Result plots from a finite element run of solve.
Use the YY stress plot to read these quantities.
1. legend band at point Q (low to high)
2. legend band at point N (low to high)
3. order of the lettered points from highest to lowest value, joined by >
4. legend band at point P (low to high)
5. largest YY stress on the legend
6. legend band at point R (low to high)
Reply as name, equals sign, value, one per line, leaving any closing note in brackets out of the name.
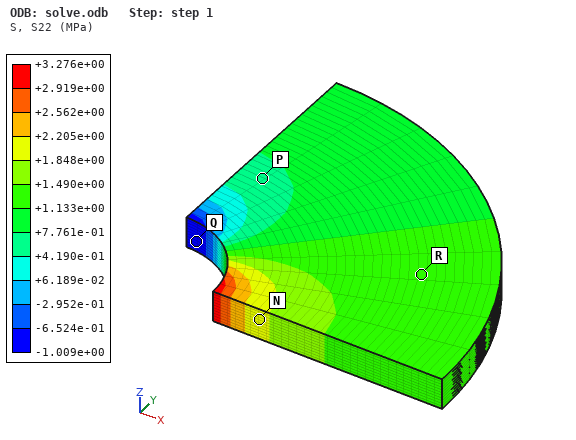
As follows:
legend band at point Q = -1.009e+00 to -6.524e-01 MPa
legend band at point N = +1.848e+00 to +2.205e+00 MPa
order of the lettered points from highest to lowest value, joined by > = N > R > P > Q
legend band at point P = +4.190e-01 to +7.761e-01 MPa
largest YY stress on the legend = +3.276e+00 MPa
legend band at point R = +1.133e+00 to +1.490e+00 MPa
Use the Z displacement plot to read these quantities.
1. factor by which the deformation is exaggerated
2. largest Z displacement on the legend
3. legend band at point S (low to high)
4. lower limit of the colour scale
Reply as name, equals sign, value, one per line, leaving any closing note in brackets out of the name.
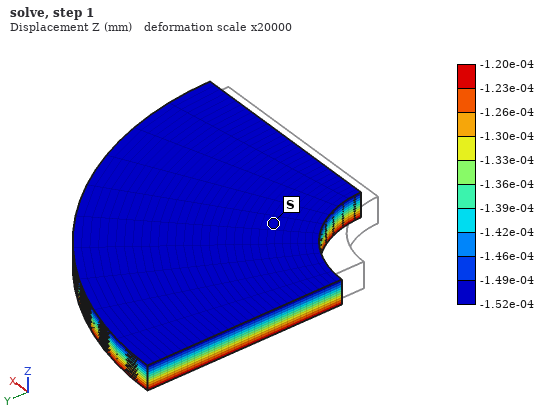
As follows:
factor by which the deformation is exaggerated = 20000
largest Z displacement on the legend = -1.20e-04 mm
legend band at point S = -1.52e-04 to -1.49e-04 mm
lower limit of the colour scale = -1.52e-04 mm
